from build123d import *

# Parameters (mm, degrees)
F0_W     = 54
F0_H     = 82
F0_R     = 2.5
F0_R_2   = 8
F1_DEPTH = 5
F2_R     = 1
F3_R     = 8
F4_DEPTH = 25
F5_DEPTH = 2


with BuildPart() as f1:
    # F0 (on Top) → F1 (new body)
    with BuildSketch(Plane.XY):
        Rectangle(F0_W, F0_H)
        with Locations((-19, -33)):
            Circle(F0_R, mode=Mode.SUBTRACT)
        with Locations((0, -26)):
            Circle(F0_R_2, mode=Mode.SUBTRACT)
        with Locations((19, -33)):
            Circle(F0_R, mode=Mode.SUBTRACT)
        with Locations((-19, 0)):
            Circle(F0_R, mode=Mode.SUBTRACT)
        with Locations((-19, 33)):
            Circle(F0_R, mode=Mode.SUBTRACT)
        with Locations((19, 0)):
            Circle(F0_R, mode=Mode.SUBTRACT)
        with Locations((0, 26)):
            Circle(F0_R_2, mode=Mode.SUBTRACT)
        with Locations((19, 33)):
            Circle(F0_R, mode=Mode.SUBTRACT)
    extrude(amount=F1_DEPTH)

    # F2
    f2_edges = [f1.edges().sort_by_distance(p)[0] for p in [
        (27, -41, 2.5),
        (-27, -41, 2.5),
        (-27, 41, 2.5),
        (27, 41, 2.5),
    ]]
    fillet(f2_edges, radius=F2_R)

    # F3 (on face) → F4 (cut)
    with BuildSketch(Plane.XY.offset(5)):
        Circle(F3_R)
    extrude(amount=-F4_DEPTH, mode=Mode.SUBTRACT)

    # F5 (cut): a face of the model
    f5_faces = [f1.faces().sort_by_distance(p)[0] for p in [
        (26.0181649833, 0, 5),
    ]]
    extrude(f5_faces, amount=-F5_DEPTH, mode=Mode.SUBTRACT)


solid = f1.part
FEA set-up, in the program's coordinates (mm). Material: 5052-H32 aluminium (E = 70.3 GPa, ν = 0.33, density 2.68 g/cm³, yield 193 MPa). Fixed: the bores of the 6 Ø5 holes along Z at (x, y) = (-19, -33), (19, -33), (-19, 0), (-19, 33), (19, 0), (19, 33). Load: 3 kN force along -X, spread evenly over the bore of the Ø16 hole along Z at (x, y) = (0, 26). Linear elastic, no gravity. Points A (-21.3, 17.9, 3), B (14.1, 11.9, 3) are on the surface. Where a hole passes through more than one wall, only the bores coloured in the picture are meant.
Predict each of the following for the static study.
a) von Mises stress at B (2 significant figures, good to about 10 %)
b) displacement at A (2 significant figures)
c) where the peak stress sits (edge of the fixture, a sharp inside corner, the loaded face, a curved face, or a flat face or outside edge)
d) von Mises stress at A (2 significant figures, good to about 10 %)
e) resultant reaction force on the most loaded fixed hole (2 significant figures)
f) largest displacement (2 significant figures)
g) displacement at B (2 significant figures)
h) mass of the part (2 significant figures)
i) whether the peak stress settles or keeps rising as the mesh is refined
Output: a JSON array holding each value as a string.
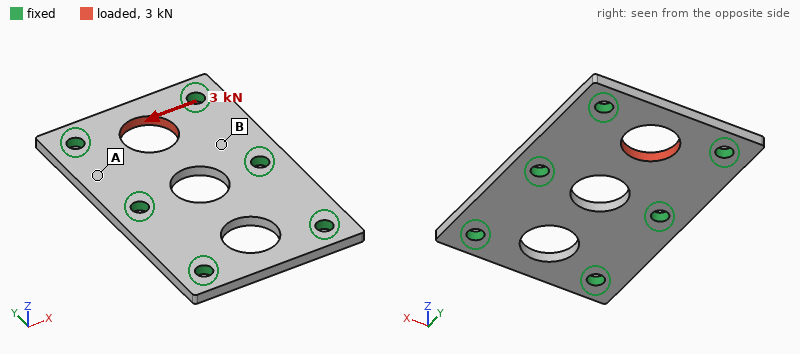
["11 MPa", "4.0 µm", "edge of the fixture", "4.6 MPa", "1.1 kN", "6.5 µm", "3.5 µm", "30 g", "keeps rising"]
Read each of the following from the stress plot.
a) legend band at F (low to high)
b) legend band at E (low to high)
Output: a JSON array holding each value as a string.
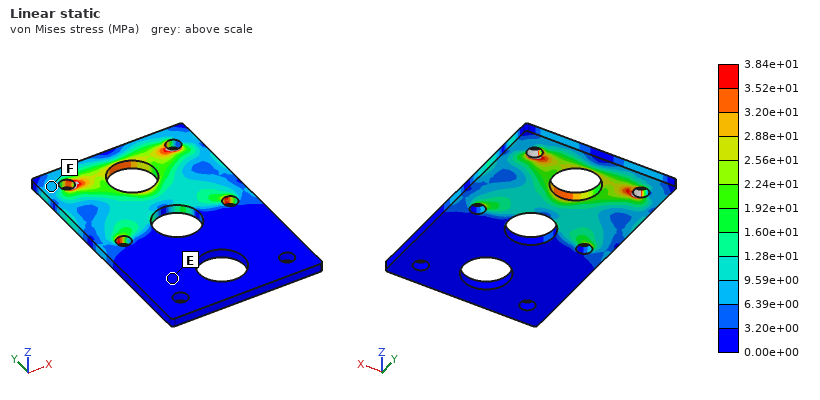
["6.39e+00 to 9.59e+00 MPa", "0.00e+00 to 3.20e+00 MPa"]
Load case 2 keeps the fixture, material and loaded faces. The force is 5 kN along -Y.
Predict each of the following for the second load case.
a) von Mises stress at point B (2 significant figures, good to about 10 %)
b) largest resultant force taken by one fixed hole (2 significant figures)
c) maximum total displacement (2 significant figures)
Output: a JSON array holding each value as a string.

["29 MPa", "1.5 kN", "26 µm"]
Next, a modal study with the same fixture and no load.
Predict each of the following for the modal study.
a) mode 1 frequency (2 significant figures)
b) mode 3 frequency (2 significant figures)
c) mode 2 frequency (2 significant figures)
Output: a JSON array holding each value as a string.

["10 kHz", "13 kHz", "10 kHz"]
